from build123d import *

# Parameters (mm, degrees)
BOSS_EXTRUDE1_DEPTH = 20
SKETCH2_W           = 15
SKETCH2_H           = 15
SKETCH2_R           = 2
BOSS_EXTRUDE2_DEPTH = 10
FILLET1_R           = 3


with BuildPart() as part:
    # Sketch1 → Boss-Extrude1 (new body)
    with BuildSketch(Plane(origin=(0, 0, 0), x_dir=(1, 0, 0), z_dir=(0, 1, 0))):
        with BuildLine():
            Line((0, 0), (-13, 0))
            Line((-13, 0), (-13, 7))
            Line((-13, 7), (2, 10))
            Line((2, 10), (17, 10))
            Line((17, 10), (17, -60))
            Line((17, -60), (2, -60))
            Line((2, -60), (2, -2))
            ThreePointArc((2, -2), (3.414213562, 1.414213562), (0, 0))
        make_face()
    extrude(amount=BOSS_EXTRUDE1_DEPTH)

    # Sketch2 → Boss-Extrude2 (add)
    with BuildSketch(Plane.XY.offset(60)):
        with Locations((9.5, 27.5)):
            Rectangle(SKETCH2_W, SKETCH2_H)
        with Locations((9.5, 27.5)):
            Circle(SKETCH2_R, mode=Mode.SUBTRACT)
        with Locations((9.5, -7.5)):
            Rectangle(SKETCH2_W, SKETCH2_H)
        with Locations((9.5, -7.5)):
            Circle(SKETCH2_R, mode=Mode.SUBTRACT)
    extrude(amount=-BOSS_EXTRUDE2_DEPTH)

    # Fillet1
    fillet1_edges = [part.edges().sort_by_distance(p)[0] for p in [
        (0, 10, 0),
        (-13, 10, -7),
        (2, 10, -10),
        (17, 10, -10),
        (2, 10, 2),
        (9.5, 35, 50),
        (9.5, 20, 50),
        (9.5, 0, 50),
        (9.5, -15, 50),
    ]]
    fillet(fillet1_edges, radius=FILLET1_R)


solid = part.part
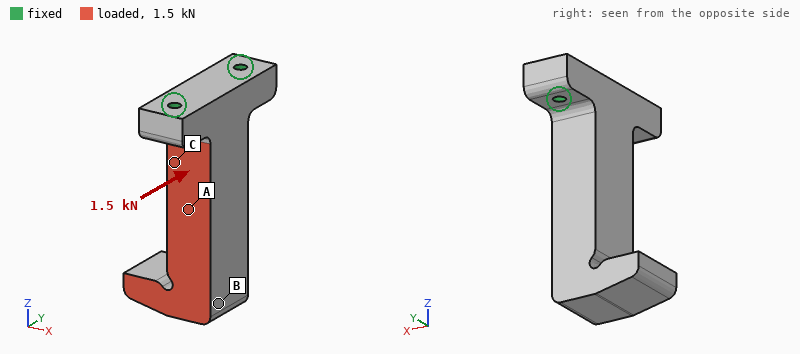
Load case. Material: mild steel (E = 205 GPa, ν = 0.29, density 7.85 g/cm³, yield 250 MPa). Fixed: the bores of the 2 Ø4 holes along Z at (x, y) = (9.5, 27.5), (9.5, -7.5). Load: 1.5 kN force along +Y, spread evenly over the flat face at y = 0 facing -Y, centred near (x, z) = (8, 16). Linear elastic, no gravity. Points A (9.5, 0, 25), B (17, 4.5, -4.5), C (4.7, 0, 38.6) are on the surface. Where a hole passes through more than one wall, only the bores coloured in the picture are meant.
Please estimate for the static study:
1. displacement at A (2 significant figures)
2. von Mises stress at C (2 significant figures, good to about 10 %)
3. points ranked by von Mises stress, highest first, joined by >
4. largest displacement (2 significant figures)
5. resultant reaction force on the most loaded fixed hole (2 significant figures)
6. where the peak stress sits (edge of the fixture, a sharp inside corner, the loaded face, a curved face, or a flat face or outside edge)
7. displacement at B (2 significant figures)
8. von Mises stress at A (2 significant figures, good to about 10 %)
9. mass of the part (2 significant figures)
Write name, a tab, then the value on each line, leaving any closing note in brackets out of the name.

displacement at A	15 µm
von Mises stress at C	35 MPa
points ranked by von Mises stress, highest first, joined by >	C > A > B
largest displacement	41 µm
resultant reaction force on the most loaded fixed hole	2.1 kN
where the peak stress sits	a curved face
displacement at B	33 µm
von Mises stress at A	20 MPa
mass of the part	220 g
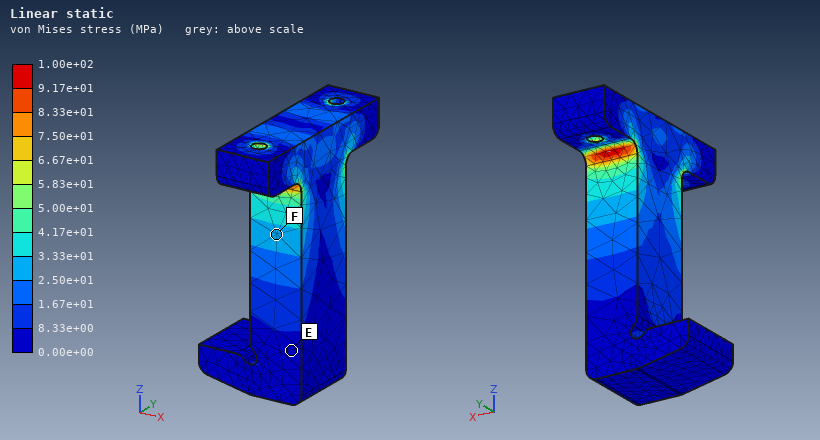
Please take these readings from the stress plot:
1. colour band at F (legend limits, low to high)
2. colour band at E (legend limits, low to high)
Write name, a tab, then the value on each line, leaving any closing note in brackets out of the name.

colour band at F	2.50e+01 to 3.33e+01 MPa
colour band at E	0.00e+00 to 8.33e+00 MPa
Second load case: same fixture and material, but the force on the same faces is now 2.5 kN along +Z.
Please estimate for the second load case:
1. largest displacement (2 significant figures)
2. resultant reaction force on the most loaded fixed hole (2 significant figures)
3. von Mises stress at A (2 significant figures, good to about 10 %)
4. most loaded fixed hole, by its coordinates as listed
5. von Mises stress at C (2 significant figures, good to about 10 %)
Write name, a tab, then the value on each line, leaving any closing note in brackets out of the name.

largest displacement	31 µm
resultant reaction force on the most loaded fixed hole	2.1 kN
von Mises stress at A	22 MPa
most loaded fixed hole, by its coordinates as listed	(9.5, -7.5)
von Mises stress at C	33 MPa
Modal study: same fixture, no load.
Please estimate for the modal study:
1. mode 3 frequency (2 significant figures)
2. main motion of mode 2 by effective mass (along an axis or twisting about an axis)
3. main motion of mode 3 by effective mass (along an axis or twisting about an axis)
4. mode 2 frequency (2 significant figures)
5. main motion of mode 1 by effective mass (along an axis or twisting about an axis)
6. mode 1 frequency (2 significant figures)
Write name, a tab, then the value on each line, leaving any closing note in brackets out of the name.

mode 3 frequency	7600 Hz
main motion of mode 2 by effective mass	along Y
main motion of mode 3 by effective mass	twisting about Z
mode 2 frequency	3000 Hz
main motion of mode 1 by effective mass	along X
mode 1 frequency	1600 Hz
